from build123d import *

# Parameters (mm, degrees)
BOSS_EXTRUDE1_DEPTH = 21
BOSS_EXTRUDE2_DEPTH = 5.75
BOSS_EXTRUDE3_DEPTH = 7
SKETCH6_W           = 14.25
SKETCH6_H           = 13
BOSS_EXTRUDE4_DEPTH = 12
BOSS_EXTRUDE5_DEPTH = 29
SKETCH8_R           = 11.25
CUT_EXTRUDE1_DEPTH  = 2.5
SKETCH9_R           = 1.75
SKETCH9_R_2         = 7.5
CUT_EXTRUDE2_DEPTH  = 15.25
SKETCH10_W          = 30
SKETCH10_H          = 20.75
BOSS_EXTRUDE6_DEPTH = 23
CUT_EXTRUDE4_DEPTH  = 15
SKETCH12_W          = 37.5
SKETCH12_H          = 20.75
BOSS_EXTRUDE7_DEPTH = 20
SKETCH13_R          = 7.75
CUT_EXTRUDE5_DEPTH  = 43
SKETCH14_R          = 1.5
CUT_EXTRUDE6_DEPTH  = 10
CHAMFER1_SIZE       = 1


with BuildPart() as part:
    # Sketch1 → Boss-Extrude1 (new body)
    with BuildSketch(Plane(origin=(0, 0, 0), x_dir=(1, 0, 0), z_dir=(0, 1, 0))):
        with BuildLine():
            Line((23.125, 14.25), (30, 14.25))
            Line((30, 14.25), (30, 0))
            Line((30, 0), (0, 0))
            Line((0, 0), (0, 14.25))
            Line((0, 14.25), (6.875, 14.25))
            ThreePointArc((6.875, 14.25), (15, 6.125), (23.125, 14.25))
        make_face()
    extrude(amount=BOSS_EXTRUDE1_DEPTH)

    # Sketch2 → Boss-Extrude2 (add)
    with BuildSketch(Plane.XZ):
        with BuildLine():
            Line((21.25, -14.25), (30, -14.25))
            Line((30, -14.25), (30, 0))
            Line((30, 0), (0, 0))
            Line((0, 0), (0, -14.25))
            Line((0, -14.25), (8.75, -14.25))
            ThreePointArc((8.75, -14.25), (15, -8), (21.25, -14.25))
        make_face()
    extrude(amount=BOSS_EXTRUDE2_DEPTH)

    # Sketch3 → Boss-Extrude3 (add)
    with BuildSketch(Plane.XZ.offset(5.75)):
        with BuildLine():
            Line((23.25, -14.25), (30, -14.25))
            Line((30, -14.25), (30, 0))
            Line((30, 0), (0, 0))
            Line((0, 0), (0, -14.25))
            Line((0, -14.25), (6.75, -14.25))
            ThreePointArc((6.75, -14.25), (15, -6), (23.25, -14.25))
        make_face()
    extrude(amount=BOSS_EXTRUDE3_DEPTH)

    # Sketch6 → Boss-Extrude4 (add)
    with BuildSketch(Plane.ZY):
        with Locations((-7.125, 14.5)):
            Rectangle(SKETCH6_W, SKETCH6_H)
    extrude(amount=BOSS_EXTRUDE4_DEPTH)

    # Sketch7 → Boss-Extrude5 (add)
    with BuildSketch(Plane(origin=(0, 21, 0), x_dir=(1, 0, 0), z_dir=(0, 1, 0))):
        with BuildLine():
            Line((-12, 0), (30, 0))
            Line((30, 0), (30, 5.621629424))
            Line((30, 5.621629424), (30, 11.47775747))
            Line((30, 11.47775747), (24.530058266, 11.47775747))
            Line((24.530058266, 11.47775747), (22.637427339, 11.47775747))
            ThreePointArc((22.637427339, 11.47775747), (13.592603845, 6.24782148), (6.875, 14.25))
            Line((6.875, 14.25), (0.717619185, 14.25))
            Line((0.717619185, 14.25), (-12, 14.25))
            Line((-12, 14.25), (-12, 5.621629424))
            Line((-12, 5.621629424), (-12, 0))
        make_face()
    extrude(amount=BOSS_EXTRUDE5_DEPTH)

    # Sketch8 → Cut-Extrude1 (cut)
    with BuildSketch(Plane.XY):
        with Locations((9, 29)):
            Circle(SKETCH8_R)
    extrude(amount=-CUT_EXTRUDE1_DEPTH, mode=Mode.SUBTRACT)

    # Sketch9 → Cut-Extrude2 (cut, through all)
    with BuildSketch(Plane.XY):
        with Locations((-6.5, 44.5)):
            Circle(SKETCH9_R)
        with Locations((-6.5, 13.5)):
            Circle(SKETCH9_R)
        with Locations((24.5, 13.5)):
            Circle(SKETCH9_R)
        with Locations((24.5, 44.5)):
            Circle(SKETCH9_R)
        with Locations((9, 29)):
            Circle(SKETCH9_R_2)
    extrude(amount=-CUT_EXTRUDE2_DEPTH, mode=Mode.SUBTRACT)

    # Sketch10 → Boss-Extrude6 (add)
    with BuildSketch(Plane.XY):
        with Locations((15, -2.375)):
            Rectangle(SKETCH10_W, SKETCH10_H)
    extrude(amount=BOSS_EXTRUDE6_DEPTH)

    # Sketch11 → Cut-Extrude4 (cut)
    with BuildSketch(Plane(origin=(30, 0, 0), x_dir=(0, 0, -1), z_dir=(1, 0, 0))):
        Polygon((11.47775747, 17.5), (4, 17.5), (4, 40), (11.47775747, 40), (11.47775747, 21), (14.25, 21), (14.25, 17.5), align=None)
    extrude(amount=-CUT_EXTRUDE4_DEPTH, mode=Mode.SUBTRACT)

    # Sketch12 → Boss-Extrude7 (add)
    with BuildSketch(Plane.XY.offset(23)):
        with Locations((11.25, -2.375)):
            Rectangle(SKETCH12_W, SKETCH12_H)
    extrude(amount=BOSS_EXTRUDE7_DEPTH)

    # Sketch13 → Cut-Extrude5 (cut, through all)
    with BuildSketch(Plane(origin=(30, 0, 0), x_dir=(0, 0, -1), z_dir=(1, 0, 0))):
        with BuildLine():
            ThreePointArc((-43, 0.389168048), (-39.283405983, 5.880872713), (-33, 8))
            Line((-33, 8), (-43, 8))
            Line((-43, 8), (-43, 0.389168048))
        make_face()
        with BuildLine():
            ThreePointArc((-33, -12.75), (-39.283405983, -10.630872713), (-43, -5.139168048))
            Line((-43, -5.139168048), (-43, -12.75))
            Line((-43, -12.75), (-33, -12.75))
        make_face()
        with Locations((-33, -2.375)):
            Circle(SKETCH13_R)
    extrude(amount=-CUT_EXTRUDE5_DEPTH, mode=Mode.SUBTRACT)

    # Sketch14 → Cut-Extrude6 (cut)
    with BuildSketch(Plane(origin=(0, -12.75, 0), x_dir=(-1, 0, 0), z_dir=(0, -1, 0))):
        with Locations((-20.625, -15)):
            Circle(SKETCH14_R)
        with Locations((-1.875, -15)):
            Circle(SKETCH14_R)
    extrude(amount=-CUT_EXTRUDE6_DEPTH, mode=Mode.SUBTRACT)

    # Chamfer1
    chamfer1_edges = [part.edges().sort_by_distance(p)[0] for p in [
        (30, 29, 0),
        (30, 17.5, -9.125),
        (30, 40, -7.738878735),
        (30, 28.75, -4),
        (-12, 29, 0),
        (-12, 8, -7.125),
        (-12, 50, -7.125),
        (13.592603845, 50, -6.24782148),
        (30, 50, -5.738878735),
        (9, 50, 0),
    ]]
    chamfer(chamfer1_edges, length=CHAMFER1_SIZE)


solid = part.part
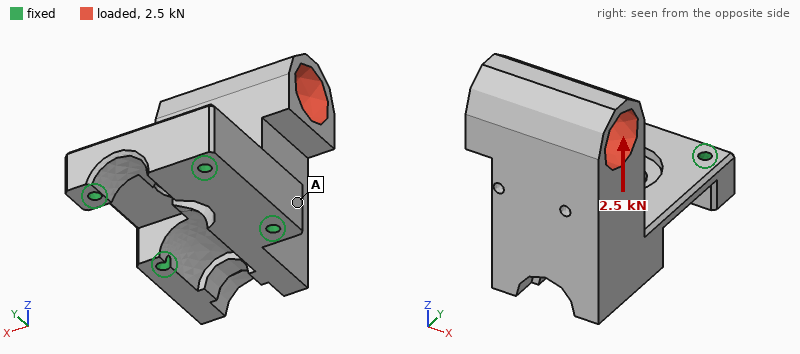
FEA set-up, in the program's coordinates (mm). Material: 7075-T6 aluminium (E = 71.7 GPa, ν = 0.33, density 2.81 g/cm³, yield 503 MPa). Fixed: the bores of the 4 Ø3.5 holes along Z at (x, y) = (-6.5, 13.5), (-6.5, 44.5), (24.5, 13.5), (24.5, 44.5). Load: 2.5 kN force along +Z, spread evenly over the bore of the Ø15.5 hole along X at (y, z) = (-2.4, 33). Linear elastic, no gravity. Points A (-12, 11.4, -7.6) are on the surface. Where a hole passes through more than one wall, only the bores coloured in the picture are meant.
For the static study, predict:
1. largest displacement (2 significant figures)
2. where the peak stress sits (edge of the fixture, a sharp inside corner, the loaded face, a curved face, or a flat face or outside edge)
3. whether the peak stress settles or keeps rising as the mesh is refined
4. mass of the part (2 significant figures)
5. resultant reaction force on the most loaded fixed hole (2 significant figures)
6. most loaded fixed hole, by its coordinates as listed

83 µm
edge of the fixture
keeps rising
120 g
1.5 kN
(-6.5, 13.5)
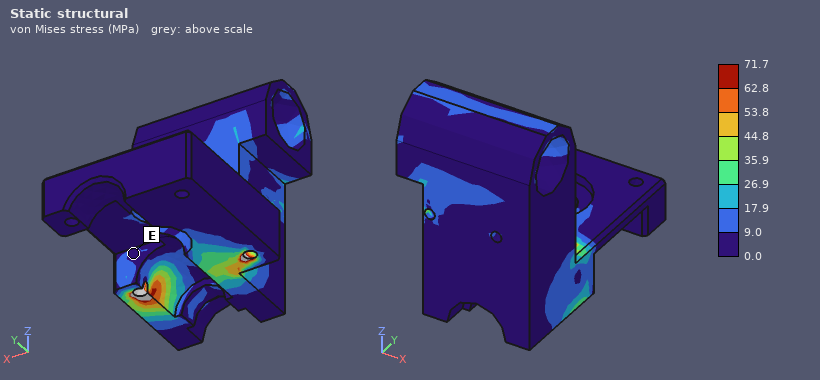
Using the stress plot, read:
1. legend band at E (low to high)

0.0 to 9.0 MPa
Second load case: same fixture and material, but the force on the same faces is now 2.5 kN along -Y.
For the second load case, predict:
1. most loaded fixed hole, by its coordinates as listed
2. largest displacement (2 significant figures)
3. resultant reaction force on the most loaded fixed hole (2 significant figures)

(24.5, 13.5)
0.29 mm
1.6 kN
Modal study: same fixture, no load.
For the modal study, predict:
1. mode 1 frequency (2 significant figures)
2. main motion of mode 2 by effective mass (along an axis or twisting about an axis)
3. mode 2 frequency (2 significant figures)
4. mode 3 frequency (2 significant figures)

3000 Hz
along X
5000 Hz
10 kHz
